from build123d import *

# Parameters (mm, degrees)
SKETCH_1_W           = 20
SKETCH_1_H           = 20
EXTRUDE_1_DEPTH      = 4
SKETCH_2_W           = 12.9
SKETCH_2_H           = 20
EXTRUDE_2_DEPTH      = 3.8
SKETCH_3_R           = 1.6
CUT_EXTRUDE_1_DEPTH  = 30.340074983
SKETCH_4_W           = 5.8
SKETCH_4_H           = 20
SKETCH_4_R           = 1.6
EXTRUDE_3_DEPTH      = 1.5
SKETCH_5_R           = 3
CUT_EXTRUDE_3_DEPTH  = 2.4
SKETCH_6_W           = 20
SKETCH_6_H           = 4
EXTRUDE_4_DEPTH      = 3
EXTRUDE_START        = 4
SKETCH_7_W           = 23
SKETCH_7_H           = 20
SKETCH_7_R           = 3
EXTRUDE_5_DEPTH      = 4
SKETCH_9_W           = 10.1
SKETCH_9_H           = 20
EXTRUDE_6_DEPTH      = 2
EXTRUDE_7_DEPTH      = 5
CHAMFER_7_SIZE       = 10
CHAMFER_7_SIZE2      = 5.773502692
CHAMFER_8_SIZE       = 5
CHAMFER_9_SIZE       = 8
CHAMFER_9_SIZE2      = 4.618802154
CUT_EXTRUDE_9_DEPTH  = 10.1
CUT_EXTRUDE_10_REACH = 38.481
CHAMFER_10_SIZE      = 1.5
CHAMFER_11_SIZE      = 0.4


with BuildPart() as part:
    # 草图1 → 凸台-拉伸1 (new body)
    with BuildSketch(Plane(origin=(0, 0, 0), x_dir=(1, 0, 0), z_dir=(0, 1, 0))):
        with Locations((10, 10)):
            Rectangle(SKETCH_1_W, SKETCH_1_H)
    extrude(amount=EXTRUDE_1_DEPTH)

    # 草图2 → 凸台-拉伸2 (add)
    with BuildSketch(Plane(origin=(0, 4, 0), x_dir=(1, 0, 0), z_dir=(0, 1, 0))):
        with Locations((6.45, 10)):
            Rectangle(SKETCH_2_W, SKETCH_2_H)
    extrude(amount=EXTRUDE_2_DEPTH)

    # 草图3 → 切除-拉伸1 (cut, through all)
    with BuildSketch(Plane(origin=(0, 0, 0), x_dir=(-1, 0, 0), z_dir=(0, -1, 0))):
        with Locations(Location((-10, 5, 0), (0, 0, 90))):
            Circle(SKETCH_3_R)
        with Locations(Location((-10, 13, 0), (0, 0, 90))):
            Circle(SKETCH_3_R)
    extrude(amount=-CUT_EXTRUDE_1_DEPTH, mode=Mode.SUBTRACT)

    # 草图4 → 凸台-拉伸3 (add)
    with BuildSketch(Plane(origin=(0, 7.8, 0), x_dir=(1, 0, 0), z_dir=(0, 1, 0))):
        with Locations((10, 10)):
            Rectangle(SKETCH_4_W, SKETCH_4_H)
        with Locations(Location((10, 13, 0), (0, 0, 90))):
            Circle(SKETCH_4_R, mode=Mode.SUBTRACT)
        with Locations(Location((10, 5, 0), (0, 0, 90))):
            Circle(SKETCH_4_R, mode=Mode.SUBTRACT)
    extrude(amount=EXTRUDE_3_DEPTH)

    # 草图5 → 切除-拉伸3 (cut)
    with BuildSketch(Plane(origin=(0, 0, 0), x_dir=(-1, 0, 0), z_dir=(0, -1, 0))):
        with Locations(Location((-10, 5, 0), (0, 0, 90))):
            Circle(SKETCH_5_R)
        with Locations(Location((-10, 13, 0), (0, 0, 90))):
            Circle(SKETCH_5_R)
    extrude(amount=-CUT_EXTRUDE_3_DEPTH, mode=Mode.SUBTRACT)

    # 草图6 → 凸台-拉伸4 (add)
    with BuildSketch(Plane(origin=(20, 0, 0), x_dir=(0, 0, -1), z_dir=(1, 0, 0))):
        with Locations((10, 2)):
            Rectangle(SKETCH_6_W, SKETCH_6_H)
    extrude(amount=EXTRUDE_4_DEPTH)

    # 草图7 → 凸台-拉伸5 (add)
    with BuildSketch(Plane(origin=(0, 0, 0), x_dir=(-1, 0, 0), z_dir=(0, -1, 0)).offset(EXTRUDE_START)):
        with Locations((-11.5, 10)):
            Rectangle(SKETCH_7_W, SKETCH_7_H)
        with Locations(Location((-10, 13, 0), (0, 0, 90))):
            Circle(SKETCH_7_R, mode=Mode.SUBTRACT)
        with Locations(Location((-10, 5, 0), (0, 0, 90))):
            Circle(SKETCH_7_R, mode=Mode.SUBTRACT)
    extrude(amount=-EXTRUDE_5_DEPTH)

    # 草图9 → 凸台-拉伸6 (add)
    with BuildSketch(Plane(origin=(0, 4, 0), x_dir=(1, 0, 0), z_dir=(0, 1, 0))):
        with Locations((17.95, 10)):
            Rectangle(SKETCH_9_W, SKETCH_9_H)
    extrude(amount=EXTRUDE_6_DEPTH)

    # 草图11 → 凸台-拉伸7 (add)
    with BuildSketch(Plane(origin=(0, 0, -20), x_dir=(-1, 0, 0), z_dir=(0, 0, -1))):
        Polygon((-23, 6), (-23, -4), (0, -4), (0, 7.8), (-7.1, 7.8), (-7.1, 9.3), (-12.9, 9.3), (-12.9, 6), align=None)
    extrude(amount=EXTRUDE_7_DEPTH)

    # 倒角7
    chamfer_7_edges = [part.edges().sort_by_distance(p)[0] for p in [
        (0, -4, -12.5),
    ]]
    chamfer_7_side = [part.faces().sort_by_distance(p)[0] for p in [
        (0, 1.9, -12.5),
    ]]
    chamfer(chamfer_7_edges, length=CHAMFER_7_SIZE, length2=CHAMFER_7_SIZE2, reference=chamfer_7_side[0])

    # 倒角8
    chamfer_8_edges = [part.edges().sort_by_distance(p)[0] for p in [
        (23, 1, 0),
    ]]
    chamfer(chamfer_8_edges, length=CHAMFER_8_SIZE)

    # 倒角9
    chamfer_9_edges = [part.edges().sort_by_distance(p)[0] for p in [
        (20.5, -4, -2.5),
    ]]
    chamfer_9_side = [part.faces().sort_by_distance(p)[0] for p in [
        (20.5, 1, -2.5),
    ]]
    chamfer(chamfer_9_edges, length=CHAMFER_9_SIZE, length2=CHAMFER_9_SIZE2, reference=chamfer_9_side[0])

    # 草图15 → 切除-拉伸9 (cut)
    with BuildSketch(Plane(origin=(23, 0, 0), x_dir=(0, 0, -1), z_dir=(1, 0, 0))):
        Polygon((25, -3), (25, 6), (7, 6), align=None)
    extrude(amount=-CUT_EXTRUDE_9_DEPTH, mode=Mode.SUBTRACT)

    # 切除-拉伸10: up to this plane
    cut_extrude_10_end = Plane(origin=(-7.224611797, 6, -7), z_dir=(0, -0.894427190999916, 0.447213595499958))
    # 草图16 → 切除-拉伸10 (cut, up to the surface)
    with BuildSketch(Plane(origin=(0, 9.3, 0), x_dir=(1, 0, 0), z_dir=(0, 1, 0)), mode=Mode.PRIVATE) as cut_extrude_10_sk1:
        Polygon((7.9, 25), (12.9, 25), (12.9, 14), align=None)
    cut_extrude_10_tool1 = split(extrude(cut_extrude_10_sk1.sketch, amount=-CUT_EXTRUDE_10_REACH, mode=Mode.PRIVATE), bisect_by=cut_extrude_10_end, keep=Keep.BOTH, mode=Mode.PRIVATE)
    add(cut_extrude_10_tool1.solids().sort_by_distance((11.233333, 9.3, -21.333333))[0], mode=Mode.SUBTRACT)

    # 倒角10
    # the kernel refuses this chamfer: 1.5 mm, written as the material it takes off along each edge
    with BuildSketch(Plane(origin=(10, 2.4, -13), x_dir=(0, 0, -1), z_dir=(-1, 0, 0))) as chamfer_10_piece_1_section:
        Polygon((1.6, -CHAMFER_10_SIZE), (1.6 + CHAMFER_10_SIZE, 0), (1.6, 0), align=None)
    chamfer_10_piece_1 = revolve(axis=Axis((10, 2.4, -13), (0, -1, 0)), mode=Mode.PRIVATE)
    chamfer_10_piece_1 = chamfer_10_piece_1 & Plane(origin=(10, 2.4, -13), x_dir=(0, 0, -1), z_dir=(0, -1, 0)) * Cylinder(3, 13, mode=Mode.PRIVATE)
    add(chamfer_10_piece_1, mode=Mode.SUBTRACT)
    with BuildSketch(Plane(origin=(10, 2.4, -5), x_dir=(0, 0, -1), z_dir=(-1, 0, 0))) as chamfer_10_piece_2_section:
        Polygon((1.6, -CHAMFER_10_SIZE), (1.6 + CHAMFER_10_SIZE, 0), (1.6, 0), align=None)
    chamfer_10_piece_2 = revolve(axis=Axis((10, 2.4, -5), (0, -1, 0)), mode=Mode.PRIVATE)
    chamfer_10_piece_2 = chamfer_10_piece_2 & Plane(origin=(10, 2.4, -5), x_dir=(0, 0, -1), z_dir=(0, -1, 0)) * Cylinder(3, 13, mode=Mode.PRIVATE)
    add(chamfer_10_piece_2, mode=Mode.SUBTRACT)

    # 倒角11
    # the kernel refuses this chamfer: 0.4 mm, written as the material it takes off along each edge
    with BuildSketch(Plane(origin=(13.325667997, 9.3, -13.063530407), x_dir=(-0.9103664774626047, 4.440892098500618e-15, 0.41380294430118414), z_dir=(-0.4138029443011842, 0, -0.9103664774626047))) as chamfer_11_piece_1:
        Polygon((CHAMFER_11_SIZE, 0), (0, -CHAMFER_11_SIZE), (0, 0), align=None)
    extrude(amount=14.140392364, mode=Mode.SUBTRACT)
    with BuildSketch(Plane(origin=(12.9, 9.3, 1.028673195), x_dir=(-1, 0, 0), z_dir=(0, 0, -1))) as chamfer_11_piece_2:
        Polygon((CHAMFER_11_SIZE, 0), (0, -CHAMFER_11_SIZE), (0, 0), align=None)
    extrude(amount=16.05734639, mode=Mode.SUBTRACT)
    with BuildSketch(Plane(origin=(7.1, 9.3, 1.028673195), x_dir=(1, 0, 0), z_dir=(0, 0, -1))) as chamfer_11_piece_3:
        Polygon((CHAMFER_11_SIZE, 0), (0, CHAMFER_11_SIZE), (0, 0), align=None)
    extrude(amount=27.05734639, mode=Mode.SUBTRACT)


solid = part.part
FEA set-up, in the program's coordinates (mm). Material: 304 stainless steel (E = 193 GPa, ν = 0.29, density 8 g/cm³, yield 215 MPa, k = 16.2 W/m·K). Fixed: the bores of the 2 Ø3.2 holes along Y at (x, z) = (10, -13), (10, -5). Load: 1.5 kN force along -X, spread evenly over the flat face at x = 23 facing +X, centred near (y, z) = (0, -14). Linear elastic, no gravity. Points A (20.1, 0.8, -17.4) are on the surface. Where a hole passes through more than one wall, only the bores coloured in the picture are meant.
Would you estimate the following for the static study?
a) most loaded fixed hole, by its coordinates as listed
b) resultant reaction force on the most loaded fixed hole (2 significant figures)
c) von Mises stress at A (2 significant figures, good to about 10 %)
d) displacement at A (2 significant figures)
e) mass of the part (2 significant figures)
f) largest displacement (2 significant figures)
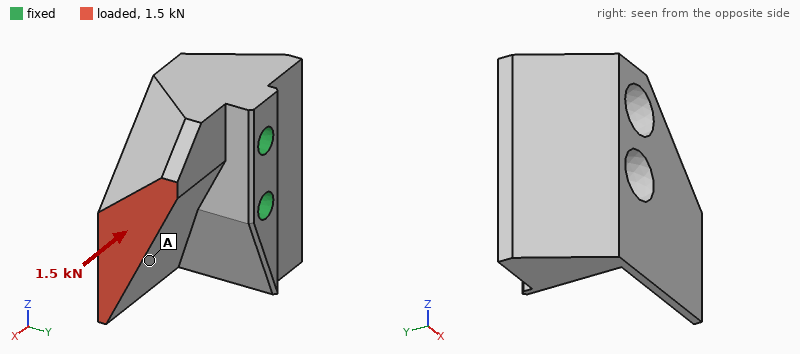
(10, -13)
1.3 kN
17 MPa
8.4 µm
31 g
13 µm
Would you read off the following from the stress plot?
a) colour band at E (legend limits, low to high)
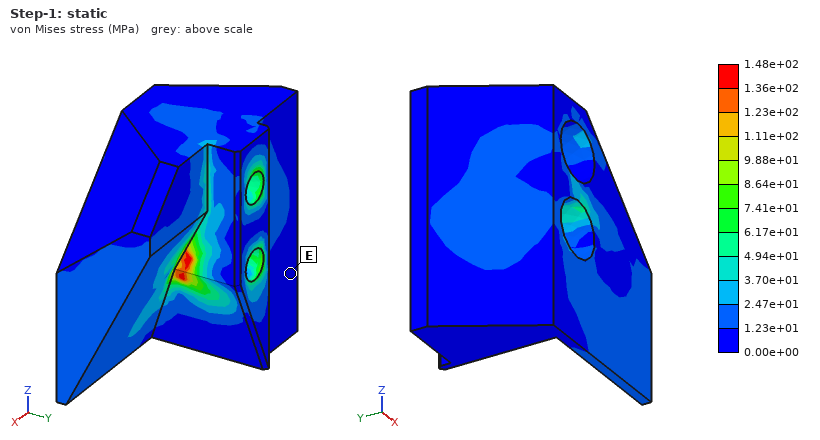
0.00e+00 to 1.23e+01 MPa
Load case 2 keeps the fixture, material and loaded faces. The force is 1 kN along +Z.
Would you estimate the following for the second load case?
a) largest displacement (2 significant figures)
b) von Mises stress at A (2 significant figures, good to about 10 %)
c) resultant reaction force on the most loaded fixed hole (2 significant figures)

12 µm
14 MPa
1.3 kN
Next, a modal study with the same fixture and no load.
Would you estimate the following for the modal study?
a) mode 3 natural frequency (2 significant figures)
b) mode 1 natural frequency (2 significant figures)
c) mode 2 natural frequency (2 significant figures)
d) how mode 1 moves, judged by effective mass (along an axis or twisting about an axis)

25 kHz
14 kHz
19 kHz
along X
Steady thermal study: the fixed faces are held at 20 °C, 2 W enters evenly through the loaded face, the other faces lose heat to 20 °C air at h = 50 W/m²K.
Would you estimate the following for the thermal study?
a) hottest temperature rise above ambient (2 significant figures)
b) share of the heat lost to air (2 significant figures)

18 K
23 %
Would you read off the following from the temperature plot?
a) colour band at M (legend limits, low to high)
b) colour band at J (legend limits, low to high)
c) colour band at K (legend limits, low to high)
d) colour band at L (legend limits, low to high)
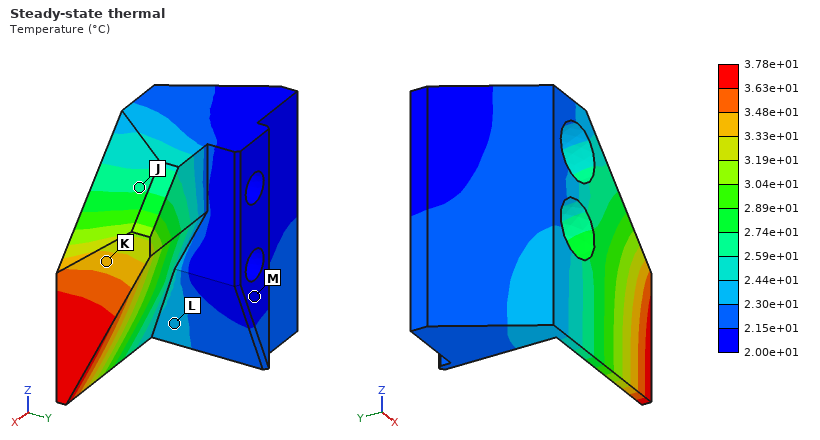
2.00e+01 to 2.15e+01 °C
2.59e+01 to 2.74e+01 °C
3.33e+01 to 3.48e+01 °C
2.30e+01 to 2.44e+01 °C
